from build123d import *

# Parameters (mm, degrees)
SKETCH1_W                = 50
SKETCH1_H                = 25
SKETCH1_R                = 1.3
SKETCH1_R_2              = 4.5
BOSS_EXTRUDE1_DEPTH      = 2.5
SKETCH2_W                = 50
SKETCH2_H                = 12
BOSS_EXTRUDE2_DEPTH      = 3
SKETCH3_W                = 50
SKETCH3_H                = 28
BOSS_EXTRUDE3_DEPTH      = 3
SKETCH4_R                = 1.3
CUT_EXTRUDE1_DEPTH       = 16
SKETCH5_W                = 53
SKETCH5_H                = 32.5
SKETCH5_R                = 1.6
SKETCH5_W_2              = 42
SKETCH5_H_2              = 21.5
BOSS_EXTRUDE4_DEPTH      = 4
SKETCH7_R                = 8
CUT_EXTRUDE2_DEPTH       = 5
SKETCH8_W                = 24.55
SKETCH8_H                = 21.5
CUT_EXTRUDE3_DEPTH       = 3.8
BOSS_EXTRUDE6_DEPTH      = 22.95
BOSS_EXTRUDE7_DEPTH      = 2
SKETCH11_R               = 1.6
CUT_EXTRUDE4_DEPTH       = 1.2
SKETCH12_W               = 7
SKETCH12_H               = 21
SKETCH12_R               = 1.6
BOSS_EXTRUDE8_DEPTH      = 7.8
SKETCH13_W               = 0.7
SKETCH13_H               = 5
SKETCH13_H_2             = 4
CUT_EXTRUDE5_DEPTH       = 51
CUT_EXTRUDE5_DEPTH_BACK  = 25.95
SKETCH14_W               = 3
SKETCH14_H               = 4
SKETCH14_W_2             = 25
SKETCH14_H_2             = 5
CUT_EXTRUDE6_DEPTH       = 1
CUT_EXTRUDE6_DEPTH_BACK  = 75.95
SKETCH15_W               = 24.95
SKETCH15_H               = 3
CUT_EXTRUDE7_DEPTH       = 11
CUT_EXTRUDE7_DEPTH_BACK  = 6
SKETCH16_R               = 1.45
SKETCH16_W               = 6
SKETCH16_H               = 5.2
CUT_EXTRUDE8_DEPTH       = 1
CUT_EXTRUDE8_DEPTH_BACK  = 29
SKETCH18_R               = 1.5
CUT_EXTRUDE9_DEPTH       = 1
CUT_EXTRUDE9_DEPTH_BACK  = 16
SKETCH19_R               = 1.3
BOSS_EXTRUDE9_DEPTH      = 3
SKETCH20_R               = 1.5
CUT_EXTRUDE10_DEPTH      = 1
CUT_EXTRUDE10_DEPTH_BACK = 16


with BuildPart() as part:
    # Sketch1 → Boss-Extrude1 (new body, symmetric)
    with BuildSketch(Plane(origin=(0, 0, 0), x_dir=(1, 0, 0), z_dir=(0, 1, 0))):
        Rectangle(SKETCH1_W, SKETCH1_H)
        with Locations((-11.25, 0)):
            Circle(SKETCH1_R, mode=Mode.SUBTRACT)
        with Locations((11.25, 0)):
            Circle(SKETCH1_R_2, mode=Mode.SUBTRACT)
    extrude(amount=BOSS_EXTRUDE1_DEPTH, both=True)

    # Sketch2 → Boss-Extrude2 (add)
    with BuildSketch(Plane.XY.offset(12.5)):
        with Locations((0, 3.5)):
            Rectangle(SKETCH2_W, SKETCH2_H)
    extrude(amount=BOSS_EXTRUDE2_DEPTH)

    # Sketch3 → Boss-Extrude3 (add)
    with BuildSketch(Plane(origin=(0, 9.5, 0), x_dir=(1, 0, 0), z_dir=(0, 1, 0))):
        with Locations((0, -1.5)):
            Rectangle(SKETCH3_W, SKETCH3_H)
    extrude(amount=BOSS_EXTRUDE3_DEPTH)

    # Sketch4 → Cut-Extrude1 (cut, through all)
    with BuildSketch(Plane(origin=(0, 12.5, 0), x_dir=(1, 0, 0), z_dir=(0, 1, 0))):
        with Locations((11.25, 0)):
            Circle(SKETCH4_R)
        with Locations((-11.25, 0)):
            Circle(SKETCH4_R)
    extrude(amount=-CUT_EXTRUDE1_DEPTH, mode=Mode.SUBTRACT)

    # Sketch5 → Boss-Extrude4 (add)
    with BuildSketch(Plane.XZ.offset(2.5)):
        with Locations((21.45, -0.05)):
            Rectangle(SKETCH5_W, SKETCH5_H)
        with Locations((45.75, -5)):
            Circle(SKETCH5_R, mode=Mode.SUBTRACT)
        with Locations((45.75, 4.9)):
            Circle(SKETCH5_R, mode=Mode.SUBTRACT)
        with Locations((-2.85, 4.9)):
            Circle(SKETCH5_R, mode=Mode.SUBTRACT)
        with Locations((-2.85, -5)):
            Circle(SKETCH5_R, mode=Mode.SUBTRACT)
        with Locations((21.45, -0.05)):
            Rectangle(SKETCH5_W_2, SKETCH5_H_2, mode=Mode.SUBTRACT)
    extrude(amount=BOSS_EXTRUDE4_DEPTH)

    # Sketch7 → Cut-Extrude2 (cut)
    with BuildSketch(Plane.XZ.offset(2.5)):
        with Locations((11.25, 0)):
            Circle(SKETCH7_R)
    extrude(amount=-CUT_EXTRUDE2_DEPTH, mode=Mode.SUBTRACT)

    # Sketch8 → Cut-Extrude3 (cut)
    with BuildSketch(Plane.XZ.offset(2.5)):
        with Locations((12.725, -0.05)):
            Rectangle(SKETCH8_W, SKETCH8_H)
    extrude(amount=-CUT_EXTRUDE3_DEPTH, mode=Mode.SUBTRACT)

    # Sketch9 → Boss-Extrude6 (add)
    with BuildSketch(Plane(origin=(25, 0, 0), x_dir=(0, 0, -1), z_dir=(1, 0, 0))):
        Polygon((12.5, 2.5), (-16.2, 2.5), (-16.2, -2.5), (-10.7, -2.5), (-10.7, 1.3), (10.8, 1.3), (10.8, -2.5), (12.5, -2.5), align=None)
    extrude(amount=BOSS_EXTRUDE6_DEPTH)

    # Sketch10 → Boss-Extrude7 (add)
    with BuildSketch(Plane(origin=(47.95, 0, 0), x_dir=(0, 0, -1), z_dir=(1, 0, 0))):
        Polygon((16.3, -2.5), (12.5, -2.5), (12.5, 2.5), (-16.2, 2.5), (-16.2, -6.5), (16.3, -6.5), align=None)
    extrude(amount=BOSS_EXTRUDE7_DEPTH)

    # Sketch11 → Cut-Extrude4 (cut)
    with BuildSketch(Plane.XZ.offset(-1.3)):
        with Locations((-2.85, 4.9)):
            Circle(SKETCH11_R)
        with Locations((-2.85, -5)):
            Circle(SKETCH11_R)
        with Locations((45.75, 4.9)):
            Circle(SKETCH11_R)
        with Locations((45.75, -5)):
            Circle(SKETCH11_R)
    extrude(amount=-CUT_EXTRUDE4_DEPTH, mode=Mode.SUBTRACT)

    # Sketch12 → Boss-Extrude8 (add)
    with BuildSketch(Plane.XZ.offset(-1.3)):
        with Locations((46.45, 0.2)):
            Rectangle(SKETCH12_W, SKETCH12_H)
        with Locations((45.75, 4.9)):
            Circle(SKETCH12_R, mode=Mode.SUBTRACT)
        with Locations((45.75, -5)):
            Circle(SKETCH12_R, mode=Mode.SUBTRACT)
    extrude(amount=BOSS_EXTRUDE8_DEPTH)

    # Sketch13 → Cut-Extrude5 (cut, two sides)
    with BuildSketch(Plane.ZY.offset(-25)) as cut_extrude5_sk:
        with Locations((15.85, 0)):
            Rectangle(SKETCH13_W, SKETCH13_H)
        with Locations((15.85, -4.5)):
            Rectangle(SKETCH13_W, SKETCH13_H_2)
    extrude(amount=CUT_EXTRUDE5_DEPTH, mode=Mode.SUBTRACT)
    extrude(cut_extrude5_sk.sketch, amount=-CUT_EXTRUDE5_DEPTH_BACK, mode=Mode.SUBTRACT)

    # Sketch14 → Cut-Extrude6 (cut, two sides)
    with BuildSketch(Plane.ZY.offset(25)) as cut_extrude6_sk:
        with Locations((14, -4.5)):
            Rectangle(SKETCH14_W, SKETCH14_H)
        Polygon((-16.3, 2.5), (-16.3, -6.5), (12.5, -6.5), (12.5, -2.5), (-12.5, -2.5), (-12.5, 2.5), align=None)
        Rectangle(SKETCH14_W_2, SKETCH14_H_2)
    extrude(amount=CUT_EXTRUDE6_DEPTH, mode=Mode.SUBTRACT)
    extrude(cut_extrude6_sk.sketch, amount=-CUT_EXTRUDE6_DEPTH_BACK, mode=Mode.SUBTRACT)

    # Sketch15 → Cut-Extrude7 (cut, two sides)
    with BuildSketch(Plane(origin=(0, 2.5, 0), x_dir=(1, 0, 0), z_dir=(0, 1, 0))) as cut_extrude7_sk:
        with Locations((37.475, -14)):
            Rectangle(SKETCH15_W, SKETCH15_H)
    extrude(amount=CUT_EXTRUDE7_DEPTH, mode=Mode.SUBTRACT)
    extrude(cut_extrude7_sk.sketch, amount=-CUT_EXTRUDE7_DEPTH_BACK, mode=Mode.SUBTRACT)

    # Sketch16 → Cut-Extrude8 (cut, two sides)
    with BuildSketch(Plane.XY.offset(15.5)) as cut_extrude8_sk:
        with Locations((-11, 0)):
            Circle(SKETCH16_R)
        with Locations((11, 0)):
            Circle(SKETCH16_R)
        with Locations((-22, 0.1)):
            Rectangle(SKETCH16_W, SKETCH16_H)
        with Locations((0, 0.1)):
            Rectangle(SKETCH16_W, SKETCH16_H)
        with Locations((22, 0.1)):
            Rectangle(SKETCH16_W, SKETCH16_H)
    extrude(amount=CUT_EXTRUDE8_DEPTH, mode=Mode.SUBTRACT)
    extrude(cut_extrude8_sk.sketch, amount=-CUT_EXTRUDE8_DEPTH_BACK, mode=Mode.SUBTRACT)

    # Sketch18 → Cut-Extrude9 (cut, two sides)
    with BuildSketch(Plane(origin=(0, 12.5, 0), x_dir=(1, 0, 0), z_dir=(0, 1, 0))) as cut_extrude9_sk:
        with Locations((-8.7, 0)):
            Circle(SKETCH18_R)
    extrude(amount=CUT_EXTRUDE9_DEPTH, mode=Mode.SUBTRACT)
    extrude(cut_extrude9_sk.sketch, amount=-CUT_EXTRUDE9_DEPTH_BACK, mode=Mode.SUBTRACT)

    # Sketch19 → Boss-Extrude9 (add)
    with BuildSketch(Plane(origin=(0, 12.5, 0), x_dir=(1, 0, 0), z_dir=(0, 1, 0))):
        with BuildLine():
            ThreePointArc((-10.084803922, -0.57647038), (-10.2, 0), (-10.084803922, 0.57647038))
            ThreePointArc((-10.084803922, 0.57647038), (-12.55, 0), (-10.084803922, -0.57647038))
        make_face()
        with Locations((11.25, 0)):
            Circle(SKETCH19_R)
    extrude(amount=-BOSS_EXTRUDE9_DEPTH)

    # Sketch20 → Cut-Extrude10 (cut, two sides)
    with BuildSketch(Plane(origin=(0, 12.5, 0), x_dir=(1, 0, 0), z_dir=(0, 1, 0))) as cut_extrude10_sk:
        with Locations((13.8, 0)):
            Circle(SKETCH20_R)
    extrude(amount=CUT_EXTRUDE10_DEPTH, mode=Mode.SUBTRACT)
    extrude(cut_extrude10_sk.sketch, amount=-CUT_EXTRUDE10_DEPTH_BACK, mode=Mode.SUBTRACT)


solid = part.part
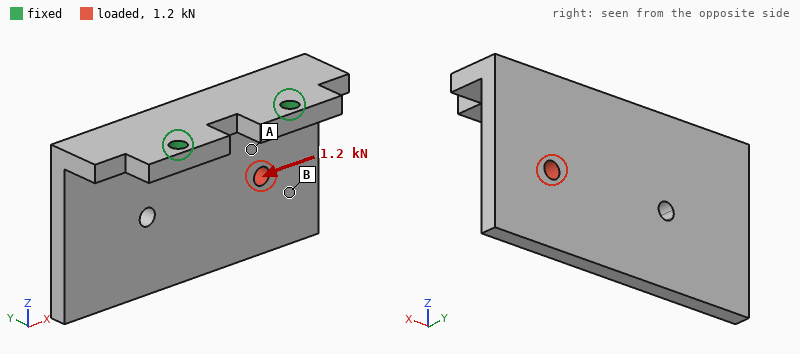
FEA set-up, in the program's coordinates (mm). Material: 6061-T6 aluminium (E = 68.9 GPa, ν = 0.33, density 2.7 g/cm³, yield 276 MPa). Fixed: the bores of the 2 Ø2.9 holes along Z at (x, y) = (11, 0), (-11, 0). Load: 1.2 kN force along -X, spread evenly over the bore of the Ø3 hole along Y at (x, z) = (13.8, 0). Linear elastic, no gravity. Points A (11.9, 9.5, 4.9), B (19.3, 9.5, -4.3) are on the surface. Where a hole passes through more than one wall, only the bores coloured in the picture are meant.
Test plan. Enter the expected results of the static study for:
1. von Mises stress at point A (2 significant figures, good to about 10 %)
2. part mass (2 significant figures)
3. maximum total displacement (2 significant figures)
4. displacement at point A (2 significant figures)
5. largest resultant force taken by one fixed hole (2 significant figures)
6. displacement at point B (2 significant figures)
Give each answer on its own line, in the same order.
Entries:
58 MPa
15 g
0.23 mm
0.092 mm
1.0 kN
0.17 mm
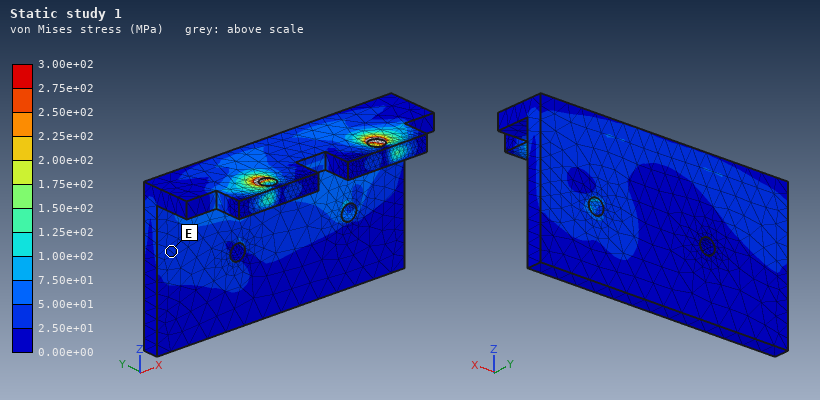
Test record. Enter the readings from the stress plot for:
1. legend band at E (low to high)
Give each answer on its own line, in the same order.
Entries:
2.50e+01 to 5.00e+01 MPa
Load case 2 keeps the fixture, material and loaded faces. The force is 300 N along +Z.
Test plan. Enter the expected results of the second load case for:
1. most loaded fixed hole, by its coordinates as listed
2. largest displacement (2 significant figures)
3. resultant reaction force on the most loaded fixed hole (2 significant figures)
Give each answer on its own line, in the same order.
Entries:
(11, 0)
0.15 mm
310 N
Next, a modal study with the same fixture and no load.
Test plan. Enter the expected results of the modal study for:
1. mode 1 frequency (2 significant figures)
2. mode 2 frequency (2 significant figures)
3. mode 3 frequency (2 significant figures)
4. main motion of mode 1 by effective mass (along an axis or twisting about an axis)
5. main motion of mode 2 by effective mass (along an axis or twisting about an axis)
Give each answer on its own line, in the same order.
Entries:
1900 Hz
3400 Hz
5300 Hz
along Y
along X
